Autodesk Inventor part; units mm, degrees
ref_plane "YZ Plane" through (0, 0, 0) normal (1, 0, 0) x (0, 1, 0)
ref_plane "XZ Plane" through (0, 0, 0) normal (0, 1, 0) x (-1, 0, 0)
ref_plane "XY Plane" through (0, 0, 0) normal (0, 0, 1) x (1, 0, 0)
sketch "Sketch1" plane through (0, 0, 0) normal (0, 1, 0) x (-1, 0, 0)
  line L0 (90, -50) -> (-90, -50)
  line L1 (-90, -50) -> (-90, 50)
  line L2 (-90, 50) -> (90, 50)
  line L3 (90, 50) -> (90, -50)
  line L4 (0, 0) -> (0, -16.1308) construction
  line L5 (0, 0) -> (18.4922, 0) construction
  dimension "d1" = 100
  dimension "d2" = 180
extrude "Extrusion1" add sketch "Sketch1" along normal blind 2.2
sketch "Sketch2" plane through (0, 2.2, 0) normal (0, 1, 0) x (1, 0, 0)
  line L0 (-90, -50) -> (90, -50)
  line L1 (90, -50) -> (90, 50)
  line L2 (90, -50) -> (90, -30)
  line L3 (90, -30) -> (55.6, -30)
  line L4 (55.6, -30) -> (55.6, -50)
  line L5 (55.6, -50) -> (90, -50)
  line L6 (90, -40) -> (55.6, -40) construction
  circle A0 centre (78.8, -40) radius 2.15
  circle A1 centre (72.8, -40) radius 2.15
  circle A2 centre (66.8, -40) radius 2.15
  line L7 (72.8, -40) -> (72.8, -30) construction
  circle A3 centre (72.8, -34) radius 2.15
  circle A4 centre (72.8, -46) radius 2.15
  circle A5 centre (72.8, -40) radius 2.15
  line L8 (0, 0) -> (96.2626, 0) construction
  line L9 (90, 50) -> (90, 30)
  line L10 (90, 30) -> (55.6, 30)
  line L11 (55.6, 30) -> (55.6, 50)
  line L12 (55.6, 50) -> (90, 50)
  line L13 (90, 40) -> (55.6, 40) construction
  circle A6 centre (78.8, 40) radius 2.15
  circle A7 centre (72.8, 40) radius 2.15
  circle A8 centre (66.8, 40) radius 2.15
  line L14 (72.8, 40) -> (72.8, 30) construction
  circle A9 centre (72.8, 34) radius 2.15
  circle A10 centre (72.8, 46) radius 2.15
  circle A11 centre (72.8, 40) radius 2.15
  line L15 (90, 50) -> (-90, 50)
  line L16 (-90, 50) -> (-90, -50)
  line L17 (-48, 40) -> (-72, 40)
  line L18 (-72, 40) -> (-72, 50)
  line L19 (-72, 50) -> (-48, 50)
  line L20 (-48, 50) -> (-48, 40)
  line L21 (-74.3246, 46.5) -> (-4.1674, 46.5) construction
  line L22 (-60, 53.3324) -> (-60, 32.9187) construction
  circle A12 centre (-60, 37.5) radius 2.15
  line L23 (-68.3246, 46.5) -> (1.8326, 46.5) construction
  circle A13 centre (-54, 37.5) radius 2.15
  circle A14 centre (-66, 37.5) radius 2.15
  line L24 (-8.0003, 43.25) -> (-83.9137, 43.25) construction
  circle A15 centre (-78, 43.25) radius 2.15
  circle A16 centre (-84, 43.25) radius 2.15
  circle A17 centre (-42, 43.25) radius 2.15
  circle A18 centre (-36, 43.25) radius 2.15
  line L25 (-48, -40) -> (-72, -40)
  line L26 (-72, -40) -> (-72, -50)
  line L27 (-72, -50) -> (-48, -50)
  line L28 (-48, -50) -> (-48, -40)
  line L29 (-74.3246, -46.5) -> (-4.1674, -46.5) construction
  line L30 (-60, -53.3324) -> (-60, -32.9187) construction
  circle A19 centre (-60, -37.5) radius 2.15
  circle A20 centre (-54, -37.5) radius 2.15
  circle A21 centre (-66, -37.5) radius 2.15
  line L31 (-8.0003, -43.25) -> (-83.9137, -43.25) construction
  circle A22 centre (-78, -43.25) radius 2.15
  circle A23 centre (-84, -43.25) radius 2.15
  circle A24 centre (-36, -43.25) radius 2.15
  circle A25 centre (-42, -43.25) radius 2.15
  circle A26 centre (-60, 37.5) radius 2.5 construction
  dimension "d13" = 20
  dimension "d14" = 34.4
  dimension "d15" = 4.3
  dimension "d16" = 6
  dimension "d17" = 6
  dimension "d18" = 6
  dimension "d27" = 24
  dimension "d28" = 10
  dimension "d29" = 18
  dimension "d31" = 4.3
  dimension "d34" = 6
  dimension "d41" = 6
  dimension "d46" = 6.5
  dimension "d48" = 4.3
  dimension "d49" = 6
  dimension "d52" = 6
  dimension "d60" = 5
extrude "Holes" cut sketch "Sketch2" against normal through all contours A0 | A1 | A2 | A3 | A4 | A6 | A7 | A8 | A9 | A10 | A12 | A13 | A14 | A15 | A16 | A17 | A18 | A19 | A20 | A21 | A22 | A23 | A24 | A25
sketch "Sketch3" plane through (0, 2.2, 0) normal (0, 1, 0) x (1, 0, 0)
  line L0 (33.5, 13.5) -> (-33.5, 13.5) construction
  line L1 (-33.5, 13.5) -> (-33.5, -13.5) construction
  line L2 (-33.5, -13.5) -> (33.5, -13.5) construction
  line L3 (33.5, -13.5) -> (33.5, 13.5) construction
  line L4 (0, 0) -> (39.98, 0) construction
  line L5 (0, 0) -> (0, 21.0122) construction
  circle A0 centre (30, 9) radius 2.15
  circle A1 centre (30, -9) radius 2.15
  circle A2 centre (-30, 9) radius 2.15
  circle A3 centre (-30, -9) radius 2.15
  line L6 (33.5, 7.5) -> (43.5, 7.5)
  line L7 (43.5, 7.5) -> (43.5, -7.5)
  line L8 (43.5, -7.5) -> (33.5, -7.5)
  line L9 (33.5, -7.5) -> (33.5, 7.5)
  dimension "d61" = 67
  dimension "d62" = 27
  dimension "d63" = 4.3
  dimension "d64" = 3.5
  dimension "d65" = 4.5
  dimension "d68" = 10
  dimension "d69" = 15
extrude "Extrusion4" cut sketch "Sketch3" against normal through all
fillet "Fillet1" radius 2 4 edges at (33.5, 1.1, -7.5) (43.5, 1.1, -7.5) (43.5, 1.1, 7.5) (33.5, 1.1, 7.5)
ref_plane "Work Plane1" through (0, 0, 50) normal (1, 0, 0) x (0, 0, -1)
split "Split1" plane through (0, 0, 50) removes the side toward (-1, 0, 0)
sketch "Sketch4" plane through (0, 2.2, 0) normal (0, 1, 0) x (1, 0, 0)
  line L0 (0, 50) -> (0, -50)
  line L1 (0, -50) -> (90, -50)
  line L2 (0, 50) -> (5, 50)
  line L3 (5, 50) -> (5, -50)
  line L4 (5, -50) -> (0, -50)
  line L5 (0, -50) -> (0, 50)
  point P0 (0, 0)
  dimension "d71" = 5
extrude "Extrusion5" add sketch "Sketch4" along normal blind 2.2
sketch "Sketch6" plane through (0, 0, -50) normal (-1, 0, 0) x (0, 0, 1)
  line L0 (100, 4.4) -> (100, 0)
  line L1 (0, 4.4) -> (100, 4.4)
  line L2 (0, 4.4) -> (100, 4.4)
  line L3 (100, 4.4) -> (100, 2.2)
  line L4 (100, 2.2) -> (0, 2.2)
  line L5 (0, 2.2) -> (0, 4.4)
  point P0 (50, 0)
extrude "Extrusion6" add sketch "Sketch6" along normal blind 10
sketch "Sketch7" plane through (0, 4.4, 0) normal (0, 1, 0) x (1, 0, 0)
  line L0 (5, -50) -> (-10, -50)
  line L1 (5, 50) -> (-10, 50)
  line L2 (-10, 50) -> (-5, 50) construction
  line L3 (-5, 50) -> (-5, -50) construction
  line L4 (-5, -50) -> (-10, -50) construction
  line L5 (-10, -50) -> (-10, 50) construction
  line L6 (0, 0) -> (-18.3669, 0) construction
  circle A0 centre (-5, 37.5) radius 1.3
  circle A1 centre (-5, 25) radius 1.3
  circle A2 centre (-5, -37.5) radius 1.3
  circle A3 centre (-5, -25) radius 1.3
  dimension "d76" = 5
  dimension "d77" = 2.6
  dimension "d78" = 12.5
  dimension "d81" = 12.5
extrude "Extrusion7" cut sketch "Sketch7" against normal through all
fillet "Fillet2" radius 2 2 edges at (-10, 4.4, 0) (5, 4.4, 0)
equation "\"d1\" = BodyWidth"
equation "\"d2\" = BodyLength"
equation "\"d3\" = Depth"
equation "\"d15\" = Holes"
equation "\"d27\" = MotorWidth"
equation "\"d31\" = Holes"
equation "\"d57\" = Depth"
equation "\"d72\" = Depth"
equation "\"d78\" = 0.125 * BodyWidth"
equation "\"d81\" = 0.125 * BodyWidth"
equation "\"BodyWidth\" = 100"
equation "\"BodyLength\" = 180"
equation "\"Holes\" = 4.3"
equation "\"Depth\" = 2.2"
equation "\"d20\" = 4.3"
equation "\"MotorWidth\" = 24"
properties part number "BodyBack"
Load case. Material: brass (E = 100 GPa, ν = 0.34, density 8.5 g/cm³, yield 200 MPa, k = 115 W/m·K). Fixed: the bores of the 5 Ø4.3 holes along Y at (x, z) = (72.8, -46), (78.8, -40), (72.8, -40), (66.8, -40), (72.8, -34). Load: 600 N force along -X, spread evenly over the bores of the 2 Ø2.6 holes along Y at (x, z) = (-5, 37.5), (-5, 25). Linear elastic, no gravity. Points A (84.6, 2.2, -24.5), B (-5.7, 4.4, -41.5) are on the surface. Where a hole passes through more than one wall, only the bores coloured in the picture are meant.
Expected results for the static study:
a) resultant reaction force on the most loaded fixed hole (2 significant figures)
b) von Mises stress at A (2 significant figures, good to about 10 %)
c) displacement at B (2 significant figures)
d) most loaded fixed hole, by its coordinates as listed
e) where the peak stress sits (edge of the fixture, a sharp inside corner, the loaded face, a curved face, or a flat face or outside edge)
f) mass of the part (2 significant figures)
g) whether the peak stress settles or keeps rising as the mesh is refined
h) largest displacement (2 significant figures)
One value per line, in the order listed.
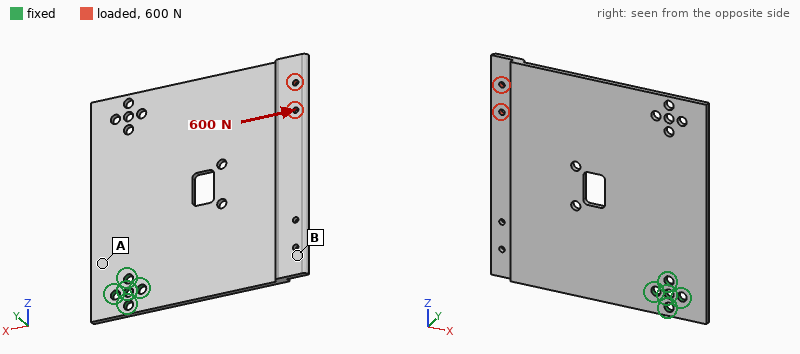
1.8 kN
39 MPa
0.52 mm
(72.8, -34)
edge of the fixture
190 g
keeps rising
0.94 mm
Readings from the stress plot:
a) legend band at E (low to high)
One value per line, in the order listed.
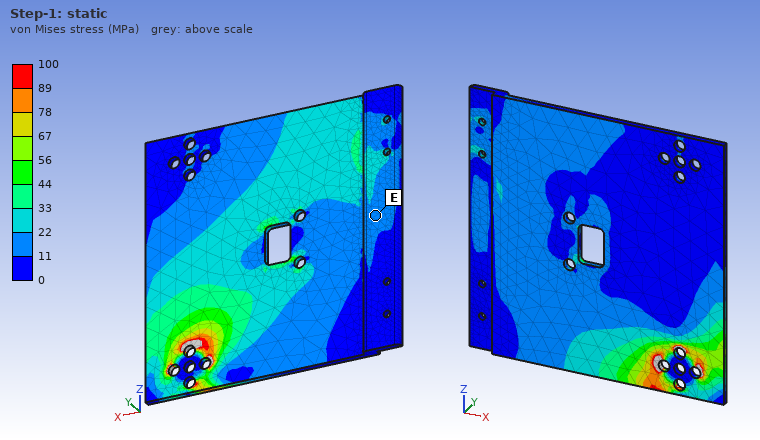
11 to 22 MPa
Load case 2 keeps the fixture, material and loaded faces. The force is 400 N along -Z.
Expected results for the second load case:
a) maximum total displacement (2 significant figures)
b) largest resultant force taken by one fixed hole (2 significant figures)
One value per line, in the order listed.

0.55 mm
1.3 kN
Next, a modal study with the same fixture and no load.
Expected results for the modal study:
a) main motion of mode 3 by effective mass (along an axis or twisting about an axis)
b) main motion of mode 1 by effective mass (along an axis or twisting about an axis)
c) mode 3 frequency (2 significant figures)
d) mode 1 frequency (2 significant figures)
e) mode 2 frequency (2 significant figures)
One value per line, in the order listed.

along Y
along Y
440 Hz
100 Hz
200 Hz
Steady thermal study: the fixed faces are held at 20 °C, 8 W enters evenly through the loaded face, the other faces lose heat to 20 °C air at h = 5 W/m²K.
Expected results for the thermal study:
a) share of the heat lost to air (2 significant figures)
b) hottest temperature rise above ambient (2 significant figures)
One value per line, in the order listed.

26 %
50 K
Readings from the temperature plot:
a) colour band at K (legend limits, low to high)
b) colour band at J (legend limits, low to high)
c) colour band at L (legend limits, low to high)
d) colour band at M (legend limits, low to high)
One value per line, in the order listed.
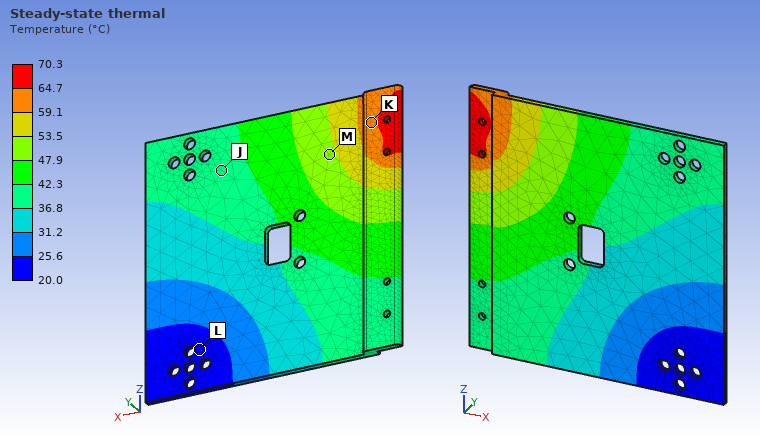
59.1 to 64.7 °C
36.8 to 42.3 °C
20.0 to 25.6 °C
47.9 to 53.5 °C
